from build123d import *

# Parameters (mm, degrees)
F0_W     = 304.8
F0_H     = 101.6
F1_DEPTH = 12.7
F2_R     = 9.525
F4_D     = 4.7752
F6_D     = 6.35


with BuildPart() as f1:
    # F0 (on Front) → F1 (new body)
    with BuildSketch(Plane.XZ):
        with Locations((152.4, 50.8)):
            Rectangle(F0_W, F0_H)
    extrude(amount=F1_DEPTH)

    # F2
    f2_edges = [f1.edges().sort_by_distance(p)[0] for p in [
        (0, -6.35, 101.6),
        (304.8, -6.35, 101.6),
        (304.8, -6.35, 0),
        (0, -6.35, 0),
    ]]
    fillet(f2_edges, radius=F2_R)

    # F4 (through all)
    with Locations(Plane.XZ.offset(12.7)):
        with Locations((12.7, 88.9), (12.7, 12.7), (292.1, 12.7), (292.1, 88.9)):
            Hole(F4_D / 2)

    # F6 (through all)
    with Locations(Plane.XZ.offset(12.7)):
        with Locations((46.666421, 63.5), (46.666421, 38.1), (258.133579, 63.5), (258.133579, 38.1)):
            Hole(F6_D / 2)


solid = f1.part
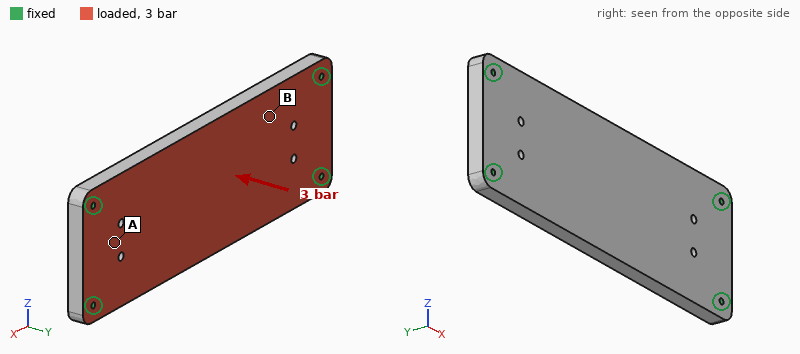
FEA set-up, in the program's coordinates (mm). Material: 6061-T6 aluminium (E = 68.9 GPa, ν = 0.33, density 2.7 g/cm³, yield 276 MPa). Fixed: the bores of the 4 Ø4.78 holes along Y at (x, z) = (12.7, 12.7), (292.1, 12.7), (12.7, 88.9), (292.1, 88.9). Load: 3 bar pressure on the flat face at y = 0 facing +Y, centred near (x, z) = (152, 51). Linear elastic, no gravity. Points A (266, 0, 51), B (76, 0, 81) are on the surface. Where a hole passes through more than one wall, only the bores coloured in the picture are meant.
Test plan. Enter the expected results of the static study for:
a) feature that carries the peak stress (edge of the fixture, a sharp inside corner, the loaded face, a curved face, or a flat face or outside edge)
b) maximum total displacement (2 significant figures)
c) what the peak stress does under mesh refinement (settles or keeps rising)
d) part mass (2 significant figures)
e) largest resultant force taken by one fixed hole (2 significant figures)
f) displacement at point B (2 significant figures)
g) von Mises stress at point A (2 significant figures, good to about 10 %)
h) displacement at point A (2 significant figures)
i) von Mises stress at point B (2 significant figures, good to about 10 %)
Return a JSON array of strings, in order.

["edge of the fixture", "0.56 mm", "keeps rising", "1.1 kg", "2.3 kN", "0.30 mm", "25 MPa", "0.11 mm", "13 MPa"]
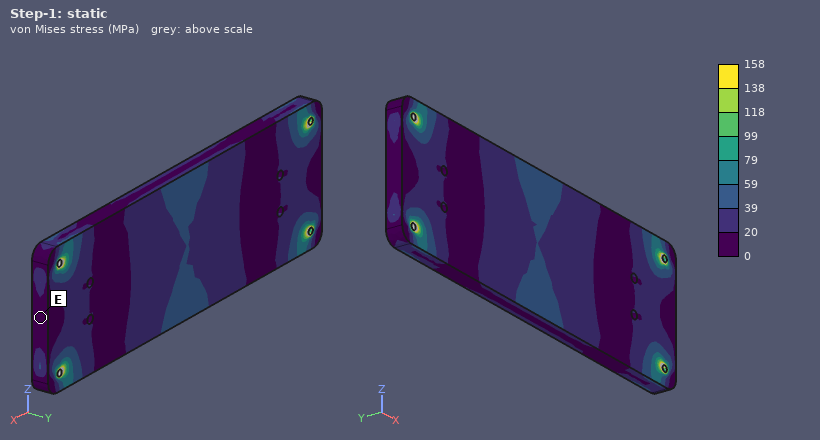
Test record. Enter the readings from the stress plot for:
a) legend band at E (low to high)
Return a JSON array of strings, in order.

["0 to 20 MPa"]
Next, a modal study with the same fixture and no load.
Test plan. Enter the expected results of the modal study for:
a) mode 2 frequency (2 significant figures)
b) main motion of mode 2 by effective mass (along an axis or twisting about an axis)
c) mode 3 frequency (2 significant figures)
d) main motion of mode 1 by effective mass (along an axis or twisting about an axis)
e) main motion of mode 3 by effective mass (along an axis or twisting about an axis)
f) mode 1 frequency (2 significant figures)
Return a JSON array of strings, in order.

["1600 Hz", "twisting about X", "2000 Hz", "along Y", "twisting about Z", "730 Hz"]
